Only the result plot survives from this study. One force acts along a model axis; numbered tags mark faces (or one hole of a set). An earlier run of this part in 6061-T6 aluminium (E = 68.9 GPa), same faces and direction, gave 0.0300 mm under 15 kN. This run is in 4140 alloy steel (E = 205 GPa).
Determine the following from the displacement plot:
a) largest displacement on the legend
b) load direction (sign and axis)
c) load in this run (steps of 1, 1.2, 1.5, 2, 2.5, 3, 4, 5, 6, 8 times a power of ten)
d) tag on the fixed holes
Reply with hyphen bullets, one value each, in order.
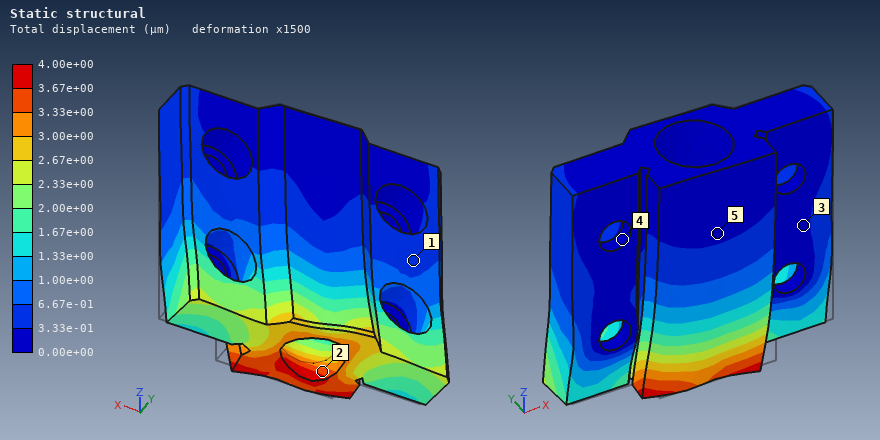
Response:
- 4.00e+00 µm
- -X
- 6 kN
- 4
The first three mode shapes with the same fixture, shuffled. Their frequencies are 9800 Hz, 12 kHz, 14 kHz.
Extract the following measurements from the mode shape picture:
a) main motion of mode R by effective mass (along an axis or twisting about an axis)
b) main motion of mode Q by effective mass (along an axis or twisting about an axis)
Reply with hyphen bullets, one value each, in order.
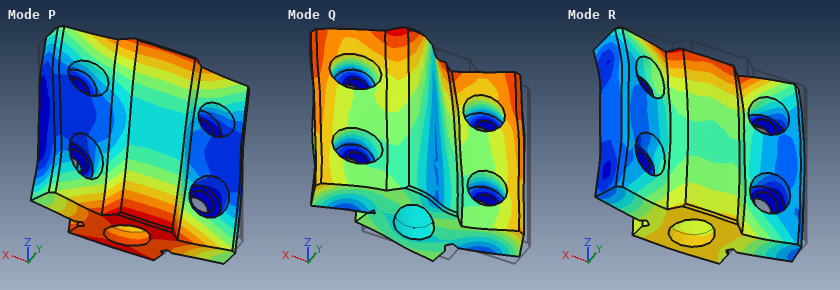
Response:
- along Y
- along X
